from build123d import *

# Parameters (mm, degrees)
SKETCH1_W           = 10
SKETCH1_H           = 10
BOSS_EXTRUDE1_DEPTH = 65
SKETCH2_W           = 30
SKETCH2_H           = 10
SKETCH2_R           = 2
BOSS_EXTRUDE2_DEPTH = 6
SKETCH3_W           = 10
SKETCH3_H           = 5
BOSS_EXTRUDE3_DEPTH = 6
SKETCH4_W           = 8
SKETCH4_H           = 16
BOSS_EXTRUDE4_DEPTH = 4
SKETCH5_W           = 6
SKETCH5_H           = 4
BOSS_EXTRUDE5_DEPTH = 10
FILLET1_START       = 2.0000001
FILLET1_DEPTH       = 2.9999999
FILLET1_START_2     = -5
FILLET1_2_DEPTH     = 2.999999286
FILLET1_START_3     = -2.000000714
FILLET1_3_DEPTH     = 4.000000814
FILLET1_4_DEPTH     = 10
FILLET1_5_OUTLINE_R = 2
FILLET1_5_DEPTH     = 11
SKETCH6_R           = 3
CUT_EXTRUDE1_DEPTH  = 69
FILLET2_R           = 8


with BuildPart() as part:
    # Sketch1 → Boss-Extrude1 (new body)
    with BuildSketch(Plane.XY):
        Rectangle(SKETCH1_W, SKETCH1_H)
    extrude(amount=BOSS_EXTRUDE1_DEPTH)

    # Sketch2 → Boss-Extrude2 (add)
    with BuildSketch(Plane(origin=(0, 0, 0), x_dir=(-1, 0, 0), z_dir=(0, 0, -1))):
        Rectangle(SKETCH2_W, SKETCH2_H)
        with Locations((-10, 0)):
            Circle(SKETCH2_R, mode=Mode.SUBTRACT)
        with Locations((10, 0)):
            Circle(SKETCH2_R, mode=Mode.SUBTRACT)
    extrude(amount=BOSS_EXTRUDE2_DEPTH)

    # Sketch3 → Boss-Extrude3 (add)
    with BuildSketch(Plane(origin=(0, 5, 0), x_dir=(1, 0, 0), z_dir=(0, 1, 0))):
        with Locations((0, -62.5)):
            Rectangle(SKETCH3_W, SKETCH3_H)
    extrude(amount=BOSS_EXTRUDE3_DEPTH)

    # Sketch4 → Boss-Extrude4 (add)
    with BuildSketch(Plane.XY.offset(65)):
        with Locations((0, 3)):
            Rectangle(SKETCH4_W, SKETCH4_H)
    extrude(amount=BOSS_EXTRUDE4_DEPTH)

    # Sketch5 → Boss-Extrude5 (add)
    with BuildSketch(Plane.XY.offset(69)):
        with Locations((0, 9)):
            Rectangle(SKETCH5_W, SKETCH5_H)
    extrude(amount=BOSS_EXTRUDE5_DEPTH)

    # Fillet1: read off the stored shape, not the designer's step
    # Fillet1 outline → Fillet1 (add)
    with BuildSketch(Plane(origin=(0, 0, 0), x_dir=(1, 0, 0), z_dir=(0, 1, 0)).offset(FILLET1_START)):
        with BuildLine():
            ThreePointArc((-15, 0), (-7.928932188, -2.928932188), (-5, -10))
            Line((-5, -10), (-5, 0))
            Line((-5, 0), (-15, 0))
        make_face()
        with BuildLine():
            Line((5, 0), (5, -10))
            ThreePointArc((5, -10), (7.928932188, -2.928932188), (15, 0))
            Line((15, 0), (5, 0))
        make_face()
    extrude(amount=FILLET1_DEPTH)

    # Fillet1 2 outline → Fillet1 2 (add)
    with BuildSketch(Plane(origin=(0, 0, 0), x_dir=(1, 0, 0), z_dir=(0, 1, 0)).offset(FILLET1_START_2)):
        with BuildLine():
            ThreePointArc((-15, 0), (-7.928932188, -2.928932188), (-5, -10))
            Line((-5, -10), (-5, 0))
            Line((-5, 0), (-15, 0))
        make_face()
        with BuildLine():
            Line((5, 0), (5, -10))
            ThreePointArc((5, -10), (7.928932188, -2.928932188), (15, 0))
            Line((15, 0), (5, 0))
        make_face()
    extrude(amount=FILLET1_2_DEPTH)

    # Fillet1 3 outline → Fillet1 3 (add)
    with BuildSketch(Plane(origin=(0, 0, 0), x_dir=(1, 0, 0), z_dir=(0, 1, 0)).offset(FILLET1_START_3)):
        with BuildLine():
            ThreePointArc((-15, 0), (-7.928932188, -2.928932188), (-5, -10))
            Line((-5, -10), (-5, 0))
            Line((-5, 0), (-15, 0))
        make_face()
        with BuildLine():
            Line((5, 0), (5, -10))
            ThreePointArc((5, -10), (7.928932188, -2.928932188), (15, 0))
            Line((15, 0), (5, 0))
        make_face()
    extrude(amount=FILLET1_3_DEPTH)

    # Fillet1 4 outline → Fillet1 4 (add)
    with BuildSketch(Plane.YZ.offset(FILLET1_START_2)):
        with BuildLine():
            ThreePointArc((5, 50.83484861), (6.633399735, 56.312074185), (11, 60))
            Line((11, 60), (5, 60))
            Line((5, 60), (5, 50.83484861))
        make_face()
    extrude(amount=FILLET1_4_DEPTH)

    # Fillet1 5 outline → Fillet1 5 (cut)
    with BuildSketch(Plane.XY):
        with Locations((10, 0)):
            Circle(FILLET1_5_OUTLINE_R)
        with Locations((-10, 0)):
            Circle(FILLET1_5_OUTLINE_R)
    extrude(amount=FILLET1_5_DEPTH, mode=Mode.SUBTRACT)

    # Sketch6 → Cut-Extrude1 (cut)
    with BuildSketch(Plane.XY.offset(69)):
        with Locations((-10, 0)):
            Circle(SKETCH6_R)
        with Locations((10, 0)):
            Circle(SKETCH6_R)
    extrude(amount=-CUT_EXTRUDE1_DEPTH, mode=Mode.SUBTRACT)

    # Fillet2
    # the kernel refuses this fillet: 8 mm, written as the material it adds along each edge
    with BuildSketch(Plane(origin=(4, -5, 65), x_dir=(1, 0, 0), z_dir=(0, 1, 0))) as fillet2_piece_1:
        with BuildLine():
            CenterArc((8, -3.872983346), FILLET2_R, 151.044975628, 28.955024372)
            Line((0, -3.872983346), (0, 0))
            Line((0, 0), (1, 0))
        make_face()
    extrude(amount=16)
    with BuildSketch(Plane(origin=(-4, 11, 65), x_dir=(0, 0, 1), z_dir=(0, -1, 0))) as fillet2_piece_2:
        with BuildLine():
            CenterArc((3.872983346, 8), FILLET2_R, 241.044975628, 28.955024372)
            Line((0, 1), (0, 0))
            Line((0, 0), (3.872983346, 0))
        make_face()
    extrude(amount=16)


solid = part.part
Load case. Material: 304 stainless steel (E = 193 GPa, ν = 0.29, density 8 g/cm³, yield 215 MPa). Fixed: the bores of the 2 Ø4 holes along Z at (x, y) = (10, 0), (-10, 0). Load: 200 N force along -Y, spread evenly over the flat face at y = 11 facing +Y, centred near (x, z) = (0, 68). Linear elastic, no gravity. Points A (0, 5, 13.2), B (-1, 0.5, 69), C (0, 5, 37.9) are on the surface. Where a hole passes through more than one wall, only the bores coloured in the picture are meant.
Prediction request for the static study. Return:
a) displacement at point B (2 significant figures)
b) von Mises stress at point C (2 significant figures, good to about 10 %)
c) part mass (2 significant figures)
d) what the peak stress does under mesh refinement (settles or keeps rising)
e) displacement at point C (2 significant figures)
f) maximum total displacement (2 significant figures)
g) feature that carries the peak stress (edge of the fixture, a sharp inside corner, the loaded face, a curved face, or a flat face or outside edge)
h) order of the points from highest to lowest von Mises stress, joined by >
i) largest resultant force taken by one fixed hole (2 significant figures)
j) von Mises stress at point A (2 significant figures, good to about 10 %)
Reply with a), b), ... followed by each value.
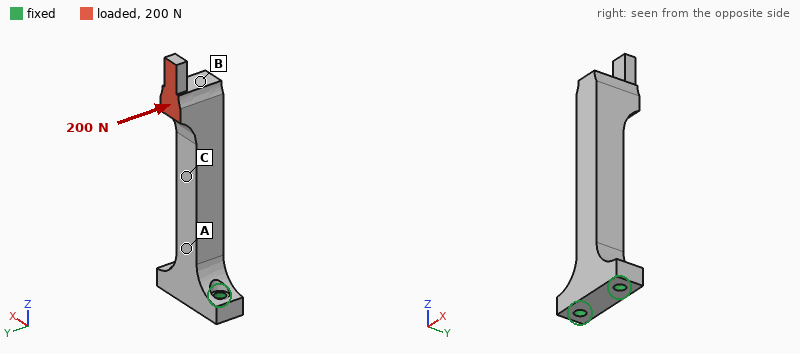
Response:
a) 0.17 mm
b) 36 MPa
c) 78 g
d) keeps rising
e) 0.072 mm
f) 0.21 mm
g) edge of the fixture
h) A > C > B
i) 100 N
j) 68 MPa
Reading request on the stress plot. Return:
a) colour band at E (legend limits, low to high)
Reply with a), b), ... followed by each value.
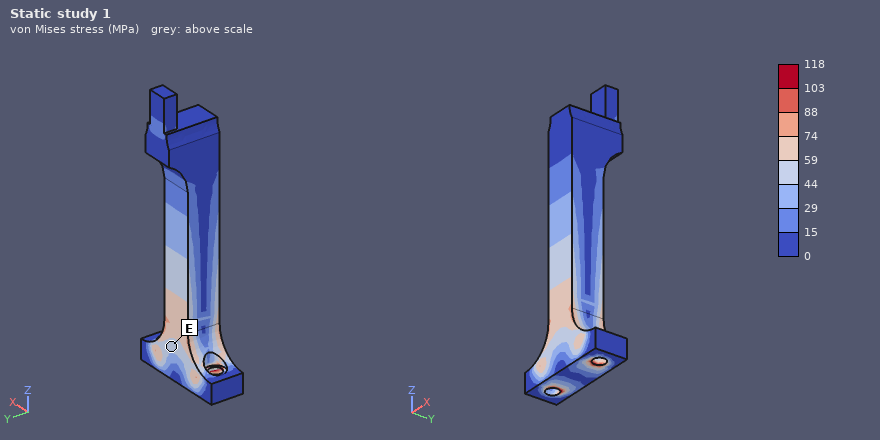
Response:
a) 44 to 59 MPa
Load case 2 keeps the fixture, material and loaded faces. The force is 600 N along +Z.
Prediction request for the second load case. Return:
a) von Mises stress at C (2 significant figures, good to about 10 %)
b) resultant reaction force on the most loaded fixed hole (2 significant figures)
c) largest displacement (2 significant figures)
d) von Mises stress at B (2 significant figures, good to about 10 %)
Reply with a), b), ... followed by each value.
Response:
a) 46 MPa
b) 320 N
c) 0.15 mm
d) 6.7 MPa
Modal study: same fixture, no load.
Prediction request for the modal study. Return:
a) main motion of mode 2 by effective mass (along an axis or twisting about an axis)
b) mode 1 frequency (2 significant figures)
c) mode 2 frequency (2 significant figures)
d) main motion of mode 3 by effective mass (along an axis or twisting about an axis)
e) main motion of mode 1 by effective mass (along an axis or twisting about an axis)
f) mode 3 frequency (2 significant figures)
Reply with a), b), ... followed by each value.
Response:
a) along X
b) 1200 Hz
c) 1500 Hz
d) along Y
e) along Y
f) 7000 Hz
